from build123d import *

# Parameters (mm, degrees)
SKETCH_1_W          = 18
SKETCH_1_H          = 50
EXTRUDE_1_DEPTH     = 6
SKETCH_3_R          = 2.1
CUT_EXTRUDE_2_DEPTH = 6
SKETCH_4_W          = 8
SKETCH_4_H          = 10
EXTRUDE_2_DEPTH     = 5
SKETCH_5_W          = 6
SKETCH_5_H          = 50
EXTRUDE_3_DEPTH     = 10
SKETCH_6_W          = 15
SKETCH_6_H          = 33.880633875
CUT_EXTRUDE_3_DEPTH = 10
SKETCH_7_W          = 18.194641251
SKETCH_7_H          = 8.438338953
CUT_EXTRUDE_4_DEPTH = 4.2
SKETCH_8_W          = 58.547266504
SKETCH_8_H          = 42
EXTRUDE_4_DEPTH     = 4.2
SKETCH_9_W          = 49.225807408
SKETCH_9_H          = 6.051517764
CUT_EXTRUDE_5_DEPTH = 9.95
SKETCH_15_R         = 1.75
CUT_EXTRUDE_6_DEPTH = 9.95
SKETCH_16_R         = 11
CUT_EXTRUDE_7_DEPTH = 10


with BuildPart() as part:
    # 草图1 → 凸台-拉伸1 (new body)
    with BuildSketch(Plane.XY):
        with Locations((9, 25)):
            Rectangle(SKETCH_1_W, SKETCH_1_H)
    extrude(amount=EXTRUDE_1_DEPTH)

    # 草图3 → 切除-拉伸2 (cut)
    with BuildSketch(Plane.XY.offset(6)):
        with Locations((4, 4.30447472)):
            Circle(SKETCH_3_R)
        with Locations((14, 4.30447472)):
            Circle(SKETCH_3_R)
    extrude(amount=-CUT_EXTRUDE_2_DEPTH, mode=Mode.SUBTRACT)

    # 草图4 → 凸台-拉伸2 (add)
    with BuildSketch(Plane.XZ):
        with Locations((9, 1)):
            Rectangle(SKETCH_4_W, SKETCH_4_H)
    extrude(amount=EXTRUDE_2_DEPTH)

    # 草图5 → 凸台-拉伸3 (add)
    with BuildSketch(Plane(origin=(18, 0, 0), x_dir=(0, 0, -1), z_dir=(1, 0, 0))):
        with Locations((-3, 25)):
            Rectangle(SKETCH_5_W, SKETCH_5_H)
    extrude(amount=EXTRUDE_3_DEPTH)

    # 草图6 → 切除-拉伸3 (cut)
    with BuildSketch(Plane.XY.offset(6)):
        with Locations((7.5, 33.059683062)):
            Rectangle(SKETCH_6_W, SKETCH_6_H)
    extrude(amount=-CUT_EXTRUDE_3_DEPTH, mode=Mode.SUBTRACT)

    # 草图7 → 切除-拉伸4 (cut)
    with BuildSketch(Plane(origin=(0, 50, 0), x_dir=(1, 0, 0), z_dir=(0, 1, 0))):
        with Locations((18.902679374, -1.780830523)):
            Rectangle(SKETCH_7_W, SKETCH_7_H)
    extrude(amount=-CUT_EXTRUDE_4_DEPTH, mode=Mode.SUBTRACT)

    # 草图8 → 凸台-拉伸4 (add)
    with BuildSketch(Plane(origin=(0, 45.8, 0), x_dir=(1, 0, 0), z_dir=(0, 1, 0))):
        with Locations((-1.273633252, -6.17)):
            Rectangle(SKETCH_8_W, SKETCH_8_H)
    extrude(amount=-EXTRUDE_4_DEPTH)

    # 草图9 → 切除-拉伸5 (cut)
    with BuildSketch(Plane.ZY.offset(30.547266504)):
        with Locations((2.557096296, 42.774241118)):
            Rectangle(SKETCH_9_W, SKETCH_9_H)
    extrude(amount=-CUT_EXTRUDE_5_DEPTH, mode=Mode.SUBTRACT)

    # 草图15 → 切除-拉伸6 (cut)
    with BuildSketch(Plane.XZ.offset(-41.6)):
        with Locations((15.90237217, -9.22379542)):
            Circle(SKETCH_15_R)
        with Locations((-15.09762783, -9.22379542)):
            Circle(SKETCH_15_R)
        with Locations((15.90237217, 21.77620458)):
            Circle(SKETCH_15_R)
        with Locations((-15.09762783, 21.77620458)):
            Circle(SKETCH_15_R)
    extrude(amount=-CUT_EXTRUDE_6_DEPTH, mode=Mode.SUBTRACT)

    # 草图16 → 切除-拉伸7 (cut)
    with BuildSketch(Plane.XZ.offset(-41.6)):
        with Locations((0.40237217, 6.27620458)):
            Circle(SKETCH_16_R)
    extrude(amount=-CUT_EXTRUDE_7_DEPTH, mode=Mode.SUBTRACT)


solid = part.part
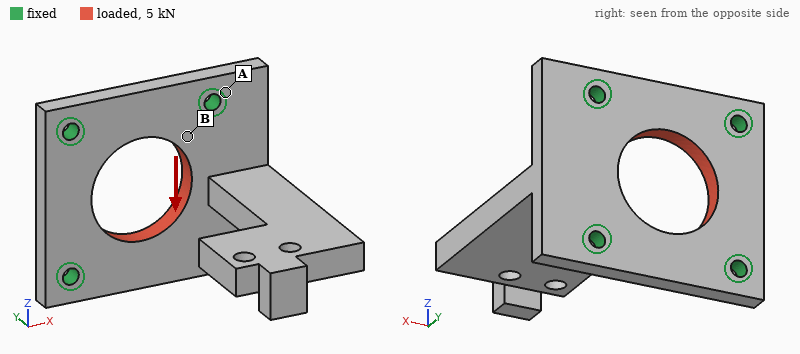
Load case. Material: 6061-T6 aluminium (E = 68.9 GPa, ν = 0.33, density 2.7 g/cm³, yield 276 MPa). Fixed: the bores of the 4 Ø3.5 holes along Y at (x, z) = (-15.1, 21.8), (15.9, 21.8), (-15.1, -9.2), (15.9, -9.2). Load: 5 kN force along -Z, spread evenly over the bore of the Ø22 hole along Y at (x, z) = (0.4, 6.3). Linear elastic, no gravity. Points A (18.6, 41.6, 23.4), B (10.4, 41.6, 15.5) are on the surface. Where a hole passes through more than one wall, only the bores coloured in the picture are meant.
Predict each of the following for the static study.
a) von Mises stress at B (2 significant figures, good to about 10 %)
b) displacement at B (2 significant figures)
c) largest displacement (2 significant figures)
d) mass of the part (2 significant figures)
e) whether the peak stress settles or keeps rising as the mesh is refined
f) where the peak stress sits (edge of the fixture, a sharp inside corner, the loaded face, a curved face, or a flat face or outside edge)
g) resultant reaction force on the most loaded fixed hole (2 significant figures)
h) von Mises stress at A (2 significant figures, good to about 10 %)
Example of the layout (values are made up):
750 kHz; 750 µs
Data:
27 MPa; 4.8 µm; 11 µm; 32 g; keeps rising; edge of the fixture; 1.3 kN; 14 MPa
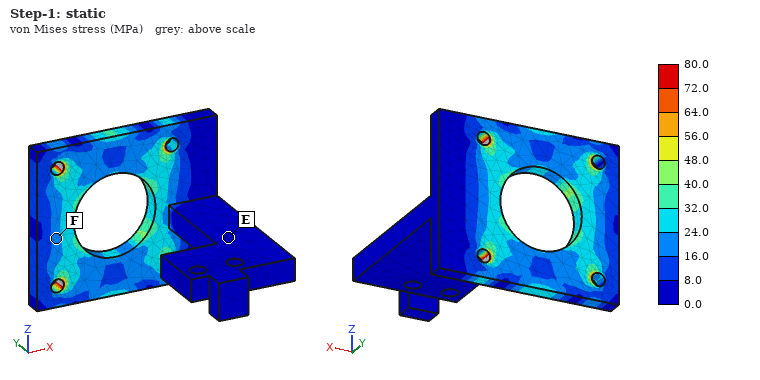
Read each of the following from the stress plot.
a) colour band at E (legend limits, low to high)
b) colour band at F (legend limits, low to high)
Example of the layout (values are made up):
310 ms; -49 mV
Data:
0.0 to 8.0 MPa; 16.0 to 24.0 MPa
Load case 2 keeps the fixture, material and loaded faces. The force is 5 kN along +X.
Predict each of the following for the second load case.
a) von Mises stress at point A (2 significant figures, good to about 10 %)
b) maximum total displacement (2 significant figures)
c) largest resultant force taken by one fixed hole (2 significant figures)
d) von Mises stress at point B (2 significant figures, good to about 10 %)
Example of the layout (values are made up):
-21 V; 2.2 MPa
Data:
8.5 MPa; 11 µm; 1.3 kN; 20 MPa
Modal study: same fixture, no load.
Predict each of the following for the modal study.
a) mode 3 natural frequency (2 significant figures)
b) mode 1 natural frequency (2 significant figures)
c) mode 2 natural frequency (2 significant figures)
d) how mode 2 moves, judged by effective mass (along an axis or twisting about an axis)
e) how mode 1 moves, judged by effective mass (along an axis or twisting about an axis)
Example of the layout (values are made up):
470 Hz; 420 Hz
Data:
5000 Hz; 1400 Hz; 1600 Hz; along X; along Z
